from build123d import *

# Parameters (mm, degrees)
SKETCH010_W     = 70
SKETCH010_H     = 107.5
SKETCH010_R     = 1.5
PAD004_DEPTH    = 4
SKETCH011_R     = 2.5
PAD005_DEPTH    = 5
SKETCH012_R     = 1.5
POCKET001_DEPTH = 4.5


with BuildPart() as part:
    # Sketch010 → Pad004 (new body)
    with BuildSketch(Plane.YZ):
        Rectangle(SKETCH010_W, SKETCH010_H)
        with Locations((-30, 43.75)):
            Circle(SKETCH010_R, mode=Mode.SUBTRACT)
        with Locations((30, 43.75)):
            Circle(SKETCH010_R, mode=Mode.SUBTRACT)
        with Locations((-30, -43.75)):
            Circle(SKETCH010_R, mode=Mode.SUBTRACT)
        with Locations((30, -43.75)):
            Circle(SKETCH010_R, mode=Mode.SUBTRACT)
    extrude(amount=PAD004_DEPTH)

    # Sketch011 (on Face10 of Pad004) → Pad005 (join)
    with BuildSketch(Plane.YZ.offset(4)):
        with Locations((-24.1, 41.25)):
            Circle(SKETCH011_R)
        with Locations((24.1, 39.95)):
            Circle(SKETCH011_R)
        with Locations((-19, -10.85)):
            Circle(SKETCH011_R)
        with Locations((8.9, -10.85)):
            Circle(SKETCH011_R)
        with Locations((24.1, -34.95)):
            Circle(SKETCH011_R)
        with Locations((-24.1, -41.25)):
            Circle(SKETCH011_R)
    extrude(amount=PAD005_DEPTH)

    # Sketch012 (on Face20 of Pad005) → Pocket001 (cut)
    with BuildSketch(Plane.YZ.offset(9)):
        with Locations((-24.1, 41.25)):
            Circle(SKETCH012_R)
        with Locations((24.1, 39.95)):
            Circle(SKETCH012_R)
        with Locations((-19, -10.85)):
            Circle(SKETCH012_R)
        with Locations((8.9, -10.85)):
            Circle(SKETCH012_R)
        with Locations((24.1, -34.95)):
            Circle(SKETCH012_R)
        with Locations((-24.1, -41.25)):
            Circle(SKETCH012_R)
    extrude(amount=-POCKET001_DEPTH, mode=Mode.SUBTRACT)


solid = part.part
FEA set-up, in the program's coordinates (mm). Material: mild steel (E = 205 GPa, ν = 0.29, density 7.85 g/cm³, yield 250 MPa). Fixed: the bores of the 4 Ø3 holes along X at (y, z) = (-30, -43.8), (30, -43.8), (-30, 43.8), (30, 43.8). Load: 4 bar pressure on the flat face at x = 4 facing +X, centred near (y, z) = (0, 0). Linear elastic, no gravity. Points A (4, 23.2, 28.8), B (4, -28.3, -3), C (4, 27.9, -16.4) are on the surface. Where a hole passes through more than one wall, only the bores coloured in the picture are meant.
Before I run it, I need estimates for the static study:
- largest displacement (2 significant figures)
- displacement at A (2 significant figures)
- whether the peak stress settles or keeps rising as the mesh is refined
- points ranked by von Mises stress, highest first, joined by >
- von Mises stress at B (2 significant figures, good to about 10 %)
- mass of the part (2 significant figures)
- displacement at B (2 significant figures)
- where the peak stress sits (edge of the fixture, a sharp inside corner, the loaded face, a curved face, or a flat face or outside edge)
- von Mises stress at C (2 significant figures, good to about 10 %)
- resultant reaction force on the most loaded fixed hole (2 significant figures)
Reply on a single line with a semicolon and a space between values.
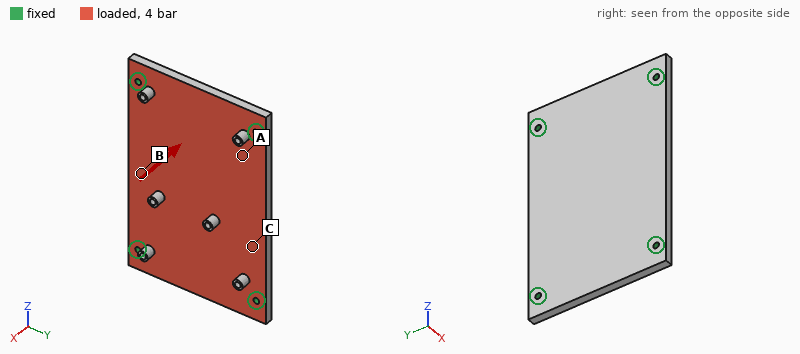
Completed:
96 µm; 39 µm; keeps rising; B > C > A; 60 MPa; 240 g; 84 µm; edge of the fixture; 42 MPa; 740 N
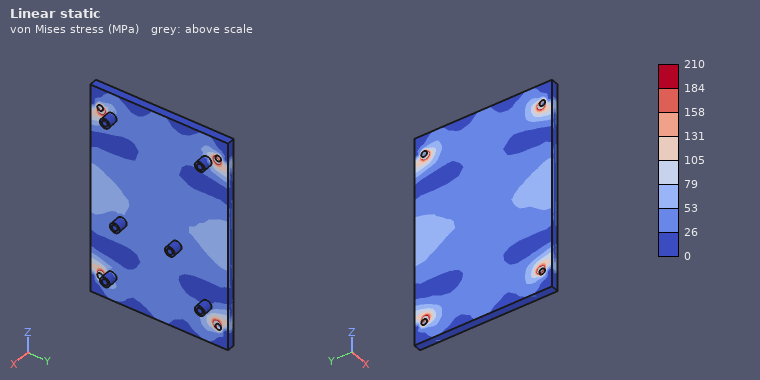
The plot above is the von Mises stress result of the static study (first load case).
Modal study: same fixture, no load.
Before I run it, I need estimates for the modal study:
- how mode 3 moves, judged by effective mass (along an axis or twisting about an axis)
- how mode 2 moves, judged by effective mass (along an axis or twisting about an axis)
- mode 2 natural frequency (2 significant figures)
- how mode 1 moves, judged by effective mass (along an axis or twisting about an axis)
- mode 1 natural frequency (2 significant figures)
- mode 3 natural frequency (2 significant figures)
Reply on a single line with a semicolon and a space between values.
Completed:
twisting about Y; twisting about Z; 3400 Hz; along X; 2100 Hz; 4900 Hz
